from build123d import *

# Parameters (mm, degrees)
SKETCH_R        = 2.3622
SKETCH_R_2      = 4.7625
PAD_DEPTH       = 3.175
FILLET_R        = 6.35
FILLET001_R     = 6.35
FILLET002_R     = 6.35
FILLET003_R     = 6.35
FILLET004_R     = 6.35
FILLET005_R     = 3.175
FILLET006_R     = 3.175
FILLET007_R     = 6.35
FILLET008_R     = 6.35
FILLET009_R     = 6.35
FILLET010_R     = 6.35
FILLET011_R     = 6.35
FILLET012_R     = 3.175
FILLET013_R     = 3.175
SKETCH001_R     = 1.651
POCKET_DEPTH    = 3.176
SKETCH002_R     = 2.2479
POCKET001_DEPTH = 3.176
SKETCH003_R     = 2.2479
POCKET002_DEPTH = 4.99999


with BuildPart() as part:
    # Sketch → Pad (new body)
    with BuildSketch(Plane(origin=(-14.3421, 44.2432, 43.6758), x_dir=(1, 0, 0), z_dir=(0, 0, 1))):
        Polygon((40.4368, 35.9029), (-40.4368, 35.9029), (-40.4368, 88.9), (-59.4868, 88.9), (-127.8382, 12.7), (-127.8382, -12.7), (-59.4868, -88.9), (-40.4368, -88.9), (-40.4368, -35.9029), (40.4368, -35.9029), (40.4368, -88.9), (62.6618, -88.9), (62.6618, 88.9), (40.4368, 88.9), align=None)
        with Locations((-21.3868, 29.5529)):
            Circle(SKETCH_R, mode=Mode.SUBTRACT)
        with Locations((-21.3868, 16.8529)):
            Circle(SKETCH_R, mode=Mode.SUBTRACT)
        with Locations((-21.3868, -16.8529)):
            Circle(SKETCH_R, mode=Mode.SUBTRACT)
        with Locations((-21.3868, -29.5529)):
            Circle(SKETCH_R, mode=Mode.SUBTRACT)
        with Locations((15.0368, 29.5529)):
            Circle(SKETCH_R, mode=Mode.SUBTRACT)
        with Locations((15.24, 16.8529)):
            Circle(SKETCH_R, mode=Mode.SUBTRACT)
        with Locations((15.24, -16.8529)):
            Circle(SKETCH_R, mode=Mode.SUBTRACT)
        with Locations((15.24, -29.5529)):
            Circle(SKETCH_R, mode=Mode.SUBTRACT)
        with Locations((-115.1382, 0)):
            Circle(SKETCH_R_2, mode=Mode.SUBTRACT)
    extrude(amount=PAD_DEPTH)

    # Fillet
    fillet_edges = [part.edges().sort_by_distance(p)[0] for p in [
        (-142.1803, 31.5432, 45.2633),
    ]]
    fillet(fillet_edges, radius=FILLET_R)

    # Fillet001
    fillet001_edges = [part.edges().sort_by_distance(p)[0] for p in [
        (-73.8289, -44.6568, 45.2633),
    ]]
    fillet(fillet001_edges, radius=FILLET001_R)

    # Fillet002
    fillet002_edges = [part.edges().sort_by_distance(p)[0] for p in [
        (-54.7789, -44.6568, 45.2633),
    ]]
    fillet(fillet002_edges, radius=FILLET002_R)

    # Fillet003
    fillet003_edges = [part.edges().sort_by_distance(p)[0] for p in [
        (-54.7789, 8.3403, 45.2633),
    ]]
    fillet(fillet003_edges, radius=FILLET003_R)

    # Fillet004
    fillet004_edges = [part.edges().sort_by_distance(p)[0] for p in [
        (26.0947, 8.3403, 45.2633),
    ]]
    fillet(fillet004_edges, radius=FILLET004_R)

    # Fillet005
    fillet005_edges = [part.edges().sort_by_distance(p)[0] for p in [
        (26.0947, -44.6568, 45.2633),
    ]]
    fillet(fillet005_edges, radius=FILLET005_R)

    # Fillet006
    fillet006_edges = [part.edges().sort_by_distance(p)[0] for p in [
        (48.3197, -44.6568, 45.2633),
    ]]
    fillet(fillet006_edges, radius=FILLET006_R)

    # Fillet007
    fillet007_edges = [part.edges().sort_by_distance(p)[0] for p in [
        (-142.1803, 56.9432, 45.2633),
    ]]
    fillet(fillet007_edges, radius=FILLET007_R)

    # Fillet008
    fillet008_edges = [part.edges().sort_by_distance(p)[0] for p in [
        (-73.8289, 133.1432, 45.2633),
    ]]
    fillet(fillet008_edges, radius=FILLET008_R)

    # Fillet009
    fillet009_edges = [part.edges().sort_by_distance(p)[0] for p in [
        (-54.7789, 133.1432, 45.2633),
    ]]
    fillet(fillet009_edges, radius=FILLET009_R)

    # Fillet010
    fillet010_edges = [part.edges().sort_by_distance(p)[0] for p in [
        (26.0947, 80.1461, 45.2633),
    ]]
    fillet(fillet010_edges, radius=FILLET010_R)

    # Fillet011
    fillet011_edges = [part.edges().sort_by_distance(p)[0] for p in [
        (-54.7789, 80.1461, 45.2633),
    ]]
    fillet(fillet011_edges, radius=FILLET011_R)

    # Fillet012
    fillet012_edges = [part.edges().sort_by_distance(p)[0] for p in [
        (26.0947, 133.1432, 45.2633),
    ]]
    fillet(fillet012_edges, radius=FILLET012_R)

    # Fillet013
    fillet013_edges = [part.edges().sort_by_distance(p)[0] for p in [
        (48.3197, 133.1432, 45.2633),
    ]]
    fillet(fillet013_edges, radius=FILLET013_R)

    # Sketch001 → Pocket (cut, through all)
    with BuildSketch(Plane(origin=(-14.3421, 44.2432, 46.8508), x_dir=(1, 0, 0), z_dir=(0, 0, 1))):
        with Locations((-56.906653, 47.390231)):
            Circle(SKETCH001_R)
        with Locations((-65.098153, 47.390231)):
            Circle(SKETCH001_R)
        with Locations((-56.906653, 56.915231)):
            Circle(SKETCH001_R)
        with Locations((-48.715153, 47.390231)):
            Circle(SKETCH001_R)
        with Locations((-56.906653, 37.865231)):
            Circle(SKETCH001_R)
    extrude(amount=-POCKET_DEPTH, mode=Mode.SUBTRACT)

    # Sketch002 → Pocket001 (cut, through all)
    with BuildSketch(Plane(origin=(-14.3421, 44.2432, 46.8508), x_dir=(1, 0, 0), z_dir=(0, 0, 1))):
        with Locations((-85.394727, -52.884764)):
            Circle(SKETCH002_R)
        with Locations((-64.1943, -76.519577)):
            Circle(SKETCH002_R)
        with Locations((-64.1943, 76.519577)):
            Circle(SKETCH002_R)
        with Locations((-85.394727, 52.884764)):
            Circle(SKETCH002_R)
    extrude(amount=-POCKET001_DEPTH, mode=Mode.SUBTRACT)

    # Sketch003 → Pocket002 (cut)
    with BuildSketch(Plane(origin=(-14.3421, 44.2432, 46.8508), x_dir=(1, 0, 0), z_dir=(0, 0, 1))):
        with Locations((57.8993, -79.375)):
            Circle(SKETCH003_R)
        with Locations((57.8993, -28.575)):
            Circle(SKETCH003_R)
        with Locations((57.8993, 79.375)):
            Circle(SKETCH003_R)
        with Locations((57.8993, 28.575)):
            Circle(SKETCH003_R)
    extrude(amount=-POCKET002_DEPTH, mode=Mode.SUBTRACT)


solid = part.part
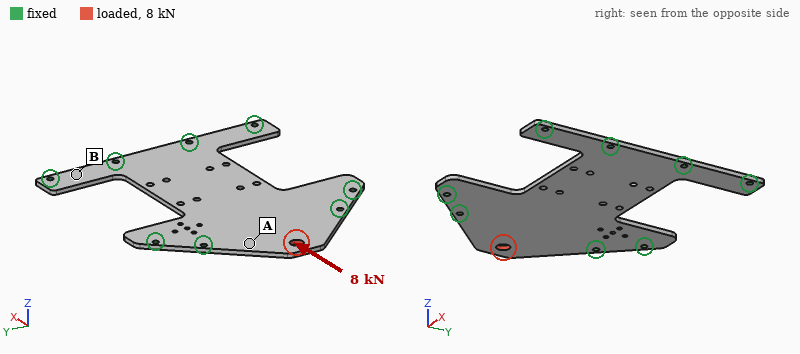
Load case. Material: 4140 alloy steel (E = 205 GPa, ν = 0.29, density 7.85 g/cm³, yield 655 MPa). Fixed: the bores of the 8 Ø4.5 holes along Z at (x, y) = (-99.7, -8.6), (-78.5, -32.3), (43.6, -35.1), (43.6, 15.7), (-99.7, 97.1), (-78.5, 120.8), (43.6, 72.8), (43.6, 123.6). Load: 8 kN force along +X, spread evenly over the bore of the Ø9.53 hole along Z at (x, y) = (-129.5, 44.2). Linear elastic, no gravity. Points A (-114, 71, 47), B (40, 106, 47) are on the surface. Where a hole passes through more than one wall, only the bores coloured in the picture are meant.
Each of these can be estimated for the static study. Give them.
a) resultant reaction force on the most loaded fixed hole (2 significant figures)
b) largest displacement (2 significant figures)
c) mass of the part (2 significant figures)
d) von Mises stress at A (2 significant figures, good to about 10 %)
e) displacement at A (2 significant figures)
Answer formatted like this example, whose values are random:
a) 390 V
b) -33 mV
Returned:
a) 2.7 kN
b) 25 µm
c) 490 g
d) 35 MPa
e) 10 µm
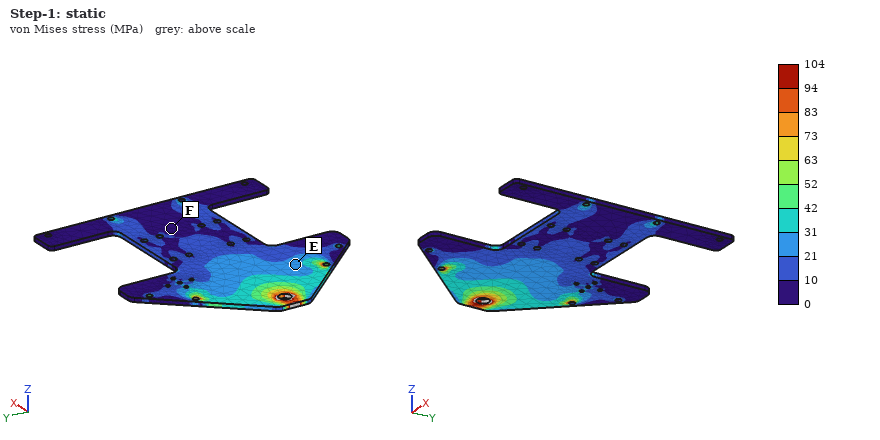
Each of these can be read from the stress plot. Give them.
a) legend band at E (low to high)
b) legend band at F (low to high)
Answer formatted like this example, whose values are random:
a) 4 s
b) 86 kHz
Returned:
a) 21 to 31 MPa
b) 0 to 10 MPa
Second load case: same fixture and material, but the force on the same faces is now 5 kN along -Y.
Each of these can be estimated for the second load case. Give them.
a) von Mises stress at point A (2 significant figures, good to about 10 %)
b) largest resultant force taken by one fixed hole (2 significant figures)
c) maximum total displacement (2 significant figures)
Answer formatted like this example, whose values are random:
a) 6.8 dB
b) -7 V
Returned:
a) 33 MPa
b) 2.4 kN
c) 17 µm
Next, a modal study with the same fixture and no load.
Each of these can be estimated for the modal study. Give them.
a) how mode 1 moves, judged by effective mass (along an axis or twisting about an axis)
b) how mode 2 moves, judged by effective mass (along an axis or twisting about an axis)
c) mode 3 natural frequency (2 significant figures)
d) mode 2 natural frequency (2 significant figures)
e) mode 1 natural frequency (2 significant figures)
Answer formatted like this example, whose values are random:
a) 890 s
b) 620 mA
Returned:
a) along Z
b) along Z
c) 1600 Hz
d) 990 Hz
e) 770 Hz
